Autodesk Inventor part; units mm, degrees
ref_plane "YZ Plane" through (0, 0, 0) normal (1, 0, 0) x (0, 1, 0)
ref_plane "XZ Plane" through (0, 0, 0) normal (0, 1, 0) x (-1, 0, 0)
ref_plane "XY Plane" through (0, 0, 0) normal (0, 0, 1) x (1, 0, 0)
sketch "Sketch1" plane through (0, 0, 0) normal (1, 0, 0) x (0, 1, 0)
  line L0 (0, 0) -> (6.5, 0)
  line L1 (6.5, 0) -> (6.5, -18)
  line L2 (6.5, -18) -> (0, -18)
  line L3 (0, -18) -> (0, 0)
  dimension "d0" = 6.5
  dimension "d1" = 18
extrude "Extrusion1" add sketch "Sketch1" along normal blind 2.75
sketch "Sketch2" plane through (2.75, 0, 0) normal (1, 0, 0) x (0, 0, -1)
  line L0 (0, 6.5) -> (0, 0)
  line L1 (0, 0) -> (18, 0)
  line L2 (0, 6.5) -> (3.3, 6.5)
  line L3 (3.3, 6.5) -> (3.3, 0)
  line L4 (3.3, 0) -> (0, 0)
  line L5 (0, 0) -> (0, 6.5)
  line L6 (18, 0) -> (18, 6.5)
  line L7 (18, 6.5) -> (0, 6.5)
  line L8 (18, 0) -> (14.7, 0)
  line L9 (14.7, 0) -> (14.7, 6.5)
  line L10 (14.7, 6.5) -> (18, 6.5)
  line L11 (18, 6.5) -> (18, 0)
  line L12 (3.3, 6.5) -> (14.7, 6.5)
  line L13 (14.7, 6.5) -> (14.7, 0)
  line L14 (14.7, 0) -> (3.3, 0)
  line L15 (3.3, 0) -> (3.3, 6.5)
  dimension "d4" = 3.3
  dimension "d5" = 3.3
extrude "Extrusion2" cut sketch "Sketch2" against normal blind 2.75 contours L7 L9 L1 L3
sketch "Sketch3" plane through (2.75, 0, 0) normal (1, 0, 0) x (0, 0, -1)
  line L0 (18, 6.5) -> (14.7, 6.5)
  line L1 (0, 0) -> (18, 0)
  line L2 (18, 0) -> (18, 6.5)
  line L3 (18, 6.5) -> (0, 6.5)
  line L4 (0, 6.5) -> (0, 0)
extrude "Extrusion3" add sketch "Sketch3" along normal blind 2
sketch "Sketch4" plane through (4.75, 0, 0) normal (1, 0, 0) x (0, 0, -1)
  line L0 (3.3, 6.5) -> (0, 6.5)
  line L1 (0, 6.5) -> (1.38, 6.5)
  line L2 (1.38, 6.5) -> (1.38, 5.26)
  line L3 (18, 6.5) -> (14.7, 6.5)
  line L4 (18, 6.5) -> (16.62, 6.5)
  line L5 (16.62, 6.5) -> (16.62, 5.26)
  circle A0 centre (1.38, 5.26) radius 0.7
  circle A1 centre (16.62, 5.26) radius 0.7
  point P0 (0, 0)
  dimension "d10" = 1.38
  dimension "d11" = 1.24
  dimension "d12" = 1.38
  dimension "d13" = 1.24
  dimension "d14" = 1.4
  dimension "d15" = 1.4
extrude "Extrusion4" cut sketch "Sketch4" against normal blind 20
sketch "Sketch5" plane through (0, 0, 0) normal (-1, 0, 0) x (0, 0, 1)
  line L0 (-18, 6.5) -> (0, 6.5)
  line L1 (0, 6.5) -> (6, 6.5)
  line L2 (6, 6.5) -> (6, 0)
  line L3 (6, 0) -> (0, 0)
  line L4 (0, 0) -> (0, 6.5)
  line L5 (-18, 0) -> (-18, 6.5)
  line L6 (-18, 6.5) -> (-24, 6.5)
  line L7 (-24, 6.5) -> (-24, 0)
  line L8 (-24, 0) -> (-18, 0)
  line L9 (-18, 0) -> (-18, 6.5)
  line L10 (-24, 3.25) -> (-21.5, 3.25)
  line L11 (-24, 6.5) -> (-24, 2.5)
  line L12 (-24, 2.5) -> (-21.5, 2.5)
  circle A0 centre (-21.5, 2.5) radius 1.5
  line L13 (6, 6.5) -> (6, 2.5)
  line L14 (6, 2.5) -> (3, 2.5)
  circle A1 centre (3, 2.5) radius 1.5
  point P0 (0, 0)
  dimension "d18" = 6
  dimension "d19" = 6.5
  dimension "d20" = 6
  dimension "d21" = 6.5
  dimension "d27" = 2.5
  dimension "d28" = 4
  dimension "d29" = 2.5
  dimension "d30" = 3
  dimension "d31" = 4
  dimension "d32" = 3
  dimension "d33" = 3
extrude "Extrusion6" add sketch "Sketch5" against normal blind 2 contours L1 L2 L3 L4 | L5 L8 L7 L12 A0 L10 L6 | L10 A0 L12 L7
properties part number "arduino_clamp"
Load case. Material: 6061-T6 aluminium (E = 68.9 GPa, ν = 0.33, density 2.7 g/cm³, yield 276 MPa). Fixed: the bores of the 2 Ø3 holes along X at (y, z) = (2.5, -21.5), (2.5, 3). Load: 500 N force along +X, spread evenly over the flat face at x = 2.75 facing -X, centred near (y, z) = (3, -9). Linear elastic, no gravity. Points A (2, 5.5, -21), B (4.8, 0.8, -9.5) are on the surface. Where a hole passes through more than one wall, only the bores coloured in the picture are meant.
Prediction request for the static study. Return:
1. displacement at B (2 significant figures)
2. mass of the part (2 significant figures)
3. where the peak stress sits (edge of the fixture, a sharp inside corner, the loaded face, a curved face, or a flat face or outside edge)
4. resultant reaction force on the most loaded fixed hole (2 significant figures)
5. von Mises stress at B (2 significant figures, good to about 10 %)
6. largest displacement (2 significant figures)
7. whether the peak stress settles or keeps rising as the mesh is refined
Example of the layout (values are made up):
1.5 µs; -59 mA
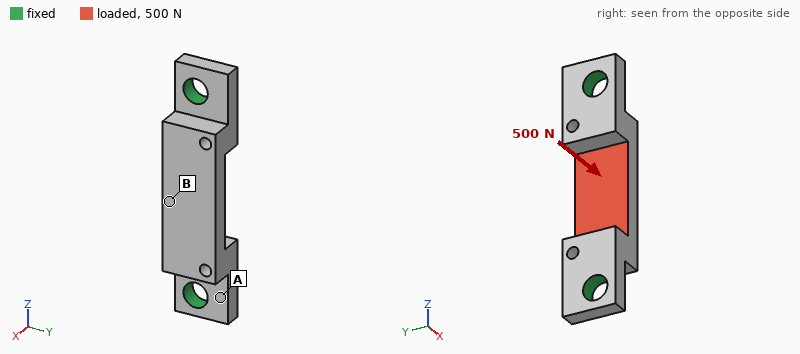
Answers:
29 µm; 1.3 g; edge of the fixture; 490 N; 130 MPa; 36 µm; keeps rising
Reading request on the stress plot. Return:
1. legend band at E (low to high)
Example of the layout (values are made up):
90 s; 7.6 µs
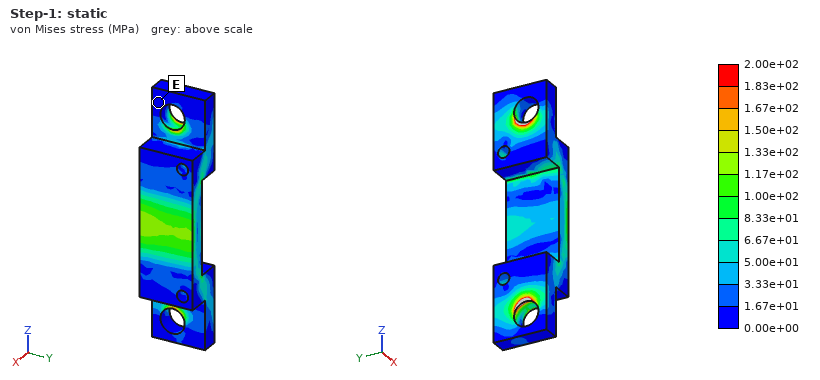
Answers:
0.00e+00 to 1.67e+01 MPa
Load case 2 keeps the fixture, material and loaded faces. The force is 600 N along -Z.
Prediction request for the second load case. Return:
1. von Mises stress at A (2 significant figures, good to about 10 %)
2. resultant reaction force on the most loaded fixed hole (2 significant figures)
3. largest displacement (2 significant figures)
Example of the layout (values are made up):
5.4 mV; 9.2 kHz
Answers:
27 MPa; 310 N; 15 µm
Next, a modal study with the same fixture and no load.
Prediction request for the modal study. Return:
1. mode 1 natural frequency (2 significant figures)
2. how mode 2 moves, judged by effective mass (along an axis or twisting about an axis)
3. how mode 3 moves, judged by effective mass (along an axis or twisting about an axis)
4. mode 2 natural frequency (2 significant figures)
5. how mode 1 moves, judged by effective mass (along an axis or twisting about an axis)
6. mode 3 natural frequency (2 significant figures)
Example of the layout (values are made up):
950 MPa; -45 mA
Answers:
26 kHz; along X; along Z; 32 kHz; along Y; 37 kHz
